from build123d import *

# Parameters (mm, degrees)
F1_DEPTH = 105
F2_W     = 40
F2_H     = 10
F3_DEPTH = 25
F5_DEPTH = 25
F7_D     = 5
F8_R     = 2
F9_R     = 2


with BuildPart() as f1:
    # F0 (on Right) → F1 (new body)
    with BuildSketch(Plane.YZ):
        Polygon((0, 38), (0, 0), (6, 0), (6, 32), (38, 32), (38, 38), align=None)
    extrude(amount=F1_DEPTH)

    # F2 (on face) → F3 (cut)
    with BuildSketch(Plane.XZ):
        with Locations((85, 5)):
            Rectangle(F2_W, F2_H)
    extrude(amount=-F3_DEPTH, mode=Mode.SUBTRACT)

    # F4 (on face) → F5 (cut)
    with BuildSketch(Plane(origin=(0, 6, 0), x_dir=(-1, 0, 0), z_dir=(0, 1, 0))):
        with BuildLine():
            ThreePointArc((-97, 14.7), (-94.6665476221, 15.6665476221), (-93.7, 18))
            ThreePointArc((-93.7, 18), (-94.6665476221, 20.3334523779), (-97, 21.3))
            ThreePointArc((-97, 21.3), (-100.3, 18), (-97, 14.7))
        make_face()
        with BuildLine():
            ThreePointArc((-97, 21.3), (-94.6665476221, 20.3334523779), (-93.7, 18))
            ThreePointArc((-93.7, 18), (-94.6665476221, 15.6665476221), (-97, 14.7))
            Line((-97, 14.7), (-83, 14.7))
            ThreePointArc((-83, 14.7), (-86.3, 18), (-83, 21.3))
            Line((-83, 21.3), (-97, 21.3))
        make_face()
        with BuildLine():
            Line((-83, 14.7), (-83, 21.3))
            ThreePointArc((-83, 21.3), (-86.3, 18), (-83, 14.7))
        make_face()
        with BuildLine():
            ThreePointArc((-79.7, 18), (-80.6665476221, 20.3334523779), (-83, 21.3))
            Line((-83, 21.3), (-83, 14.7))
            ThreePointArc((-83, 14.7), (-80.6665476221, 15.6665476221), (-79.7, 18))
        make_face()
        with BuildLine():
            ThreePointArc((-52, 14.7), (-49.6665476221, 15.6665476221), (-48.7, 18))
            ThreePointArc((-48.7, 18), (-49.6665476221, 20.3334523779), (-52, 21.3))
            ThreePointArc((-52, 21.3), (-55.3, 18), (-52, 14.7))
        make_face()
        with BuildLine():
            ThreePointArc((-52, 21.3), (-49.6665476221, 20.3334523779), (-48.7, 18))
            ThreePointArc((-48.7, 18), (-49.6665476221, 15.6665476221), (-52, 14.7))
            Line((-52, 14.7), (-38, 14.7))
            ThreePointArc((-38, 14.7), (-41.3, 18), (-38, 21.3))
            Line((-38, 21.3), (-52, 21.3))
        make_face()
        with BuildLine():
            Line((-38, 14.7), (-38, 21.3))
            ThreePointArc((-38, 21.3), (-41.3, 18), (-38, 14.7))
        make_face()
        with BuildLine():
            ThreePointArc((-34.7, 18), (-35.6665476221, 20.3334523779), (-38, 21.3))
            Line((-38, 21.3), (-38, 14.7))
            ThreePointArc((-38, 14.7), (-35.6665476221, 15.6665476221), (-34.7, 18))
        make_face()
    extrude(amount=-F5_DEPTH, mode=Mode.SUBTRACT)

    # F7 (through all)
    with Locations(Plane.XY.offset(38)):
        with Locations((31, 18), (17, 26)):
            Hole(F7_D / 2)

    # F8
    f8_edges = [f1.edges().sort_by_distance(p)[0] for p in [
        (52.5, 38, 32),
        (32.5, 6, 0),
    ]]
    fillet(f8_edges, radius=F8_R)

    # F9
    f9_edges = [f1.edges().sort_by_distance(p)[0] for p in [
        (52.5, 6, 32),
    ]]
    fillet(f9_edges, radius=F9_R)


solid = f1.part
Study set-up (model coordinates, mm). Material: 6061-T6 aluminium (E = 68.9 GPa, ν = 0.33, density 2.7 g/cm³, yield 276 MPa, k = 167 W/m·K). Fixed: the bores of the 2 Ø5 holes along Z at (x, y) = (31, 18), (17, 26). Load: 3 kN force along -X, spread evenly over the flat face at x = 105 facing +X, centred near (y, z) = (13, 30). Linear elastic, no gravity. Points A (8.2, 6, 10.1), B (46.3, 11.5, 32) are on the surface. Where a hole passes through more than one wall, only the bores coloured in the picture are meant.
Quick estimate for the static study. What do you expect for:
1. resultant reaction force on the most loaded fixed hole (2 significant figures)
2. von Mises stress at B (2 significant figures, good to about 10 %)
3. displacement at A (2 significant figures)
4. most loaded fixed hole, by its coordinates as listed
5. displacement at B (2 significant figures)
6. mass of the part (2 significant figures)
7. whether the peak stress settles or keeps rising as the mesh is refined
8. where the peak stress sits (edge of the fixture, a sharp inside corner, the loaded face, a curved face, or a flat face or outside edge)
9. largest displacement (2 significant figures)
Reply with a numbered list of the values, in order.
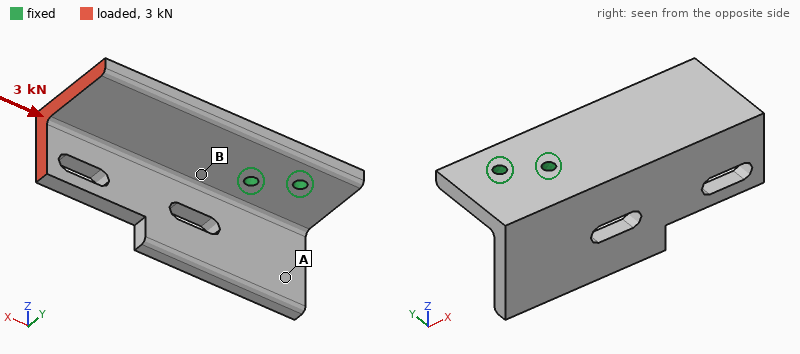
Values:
1. 2.8 kN
2. 17 MPa
3. 0.061 mm
4. (31, 18)
5. 0.023 mm
6. 110 g
7. keeps rising
8. edge of the fixture
9. 0.14 mm
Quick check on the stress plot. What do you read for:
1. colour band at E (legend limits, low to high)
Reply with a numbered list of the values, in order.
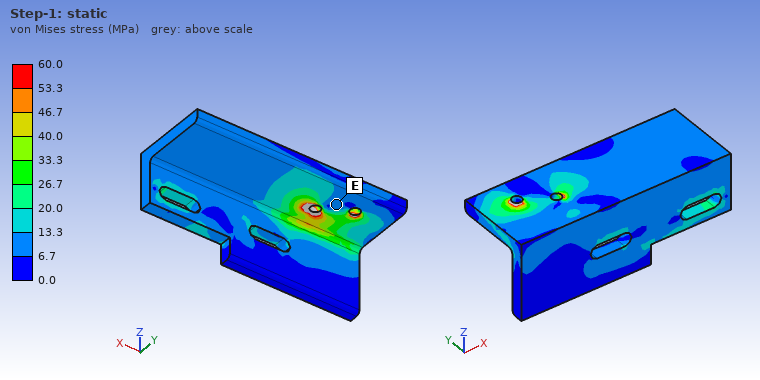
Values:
1. 6.7 to 13.3 MPa
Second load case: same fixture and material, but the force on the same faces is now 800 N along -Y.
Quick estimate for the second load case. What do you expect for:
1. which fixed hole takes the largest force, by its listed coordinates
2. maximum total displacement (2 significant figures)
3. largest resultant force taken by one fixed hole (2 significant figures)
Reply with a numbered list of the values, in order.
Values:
1. (31, 18)
2. 0.23 mm
3. 3.5 kN
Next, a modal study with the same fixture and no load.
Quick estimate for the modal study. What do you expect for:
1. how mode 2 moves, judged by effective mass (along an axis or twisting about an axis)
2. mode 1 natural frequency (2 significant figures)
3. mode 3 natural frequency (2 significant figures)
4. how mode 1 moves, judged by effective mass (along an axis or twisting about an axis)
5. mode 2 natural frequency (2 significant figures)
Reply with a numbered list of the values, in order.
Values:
1. along Y
2. 1200 Hz
3. 2800 Hz
4. along Z
5. 1900 Hz
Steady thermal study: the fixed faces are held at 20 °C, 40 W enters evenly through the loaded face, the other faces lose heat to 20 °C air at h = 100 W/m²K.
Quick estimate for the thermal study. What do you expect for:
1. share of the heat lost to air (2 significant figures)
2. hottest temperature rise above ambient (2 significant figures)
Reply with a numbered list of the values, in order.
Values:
1. 51 %
2. 41 K
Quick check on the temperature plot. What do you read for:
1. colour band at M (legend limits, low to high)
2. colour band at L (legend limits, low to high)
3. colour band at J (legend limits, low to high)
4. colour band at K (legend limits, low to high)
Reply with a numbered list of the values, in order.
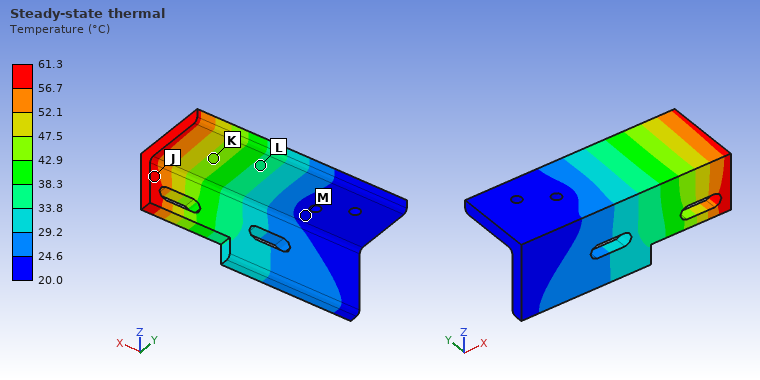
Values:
1. 20.0 to 24.6 °C
2. 33.8 to 38.3 °C
3. 56.7 to 61.3 °C
4. 42.9 to 47.5 °C
